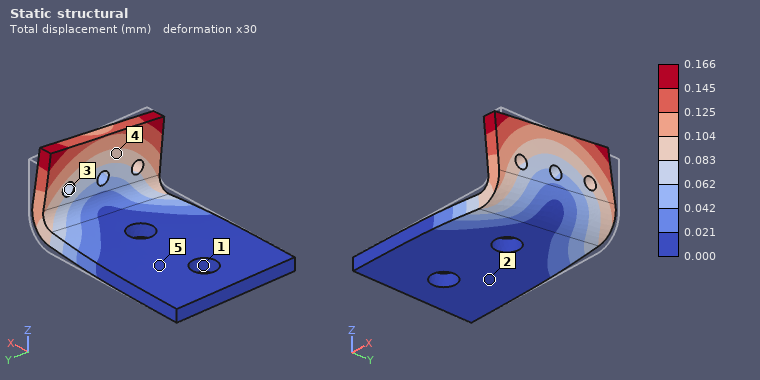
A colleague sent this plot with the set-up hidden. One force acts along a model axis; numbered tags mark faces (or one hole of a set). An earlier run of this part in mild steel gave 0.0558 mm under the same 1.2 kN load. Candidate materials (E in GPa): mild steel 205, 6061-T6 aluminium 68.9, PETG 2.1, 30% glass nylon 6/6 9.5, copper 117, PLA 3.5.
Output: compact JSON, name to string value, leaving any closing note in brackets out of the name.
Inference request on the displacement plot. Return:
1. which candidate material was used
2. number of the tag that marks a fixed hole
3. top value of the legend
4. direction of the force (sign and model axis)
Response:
{"which candidate material was used": "6061-T6 aluminium", "number of the tag that marks a fixed hole": "1", "top value of the legend": "0.166 mm", "direction of the force": "-Y"}
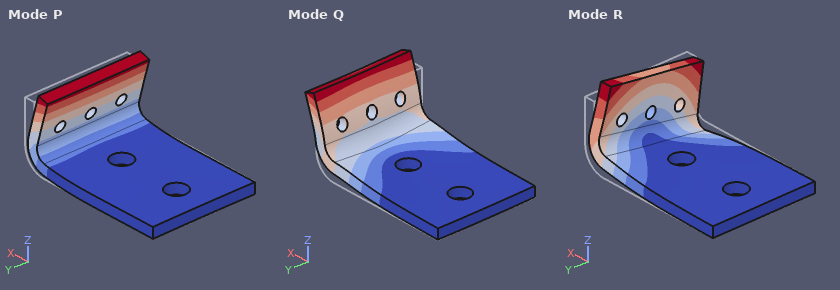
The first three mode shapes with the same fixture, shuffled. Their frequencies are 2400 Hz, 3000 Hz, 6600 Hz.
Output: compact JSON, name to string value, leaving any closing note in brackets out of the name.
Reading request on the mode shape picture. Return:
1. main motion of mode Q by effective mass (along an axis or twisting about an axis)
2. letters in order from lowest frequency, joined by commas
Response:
{"main motion of mode Q by effective mass": "along Z", "letters in order from lowest frequency, joined by commas": "P, R, Q"}
